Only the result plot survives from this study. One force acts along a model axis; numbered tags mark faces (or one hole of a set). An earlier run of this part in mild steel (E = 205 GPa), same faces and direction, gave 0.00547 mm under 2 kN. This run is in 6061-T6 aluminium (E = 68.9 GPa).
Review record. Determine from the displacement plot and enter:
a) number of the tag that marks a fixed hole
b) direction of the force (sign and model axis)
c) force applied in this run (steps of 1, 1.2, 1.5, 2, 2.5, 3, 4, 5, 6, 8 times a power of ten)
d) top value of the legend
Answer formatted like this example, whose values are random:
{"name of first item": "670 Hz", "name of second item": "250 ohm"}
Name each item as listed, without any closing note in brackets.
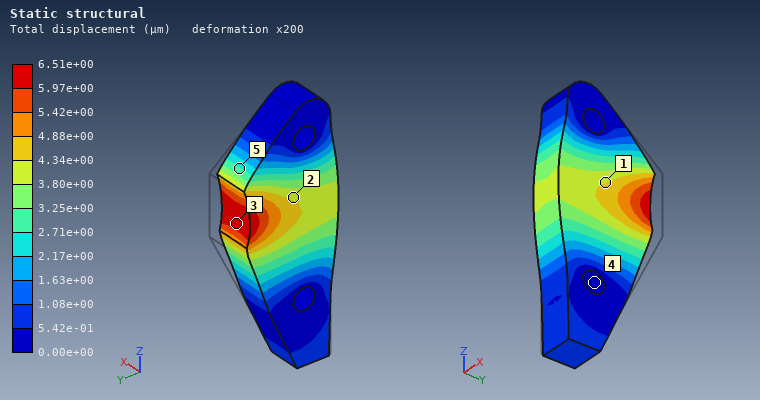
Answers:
{"number of the tag that marks a fixed hole": "4", "direction of the force": "-Y", "force applied in this run": "800 N", "top value of the legend": "6.51e+00 µm"}
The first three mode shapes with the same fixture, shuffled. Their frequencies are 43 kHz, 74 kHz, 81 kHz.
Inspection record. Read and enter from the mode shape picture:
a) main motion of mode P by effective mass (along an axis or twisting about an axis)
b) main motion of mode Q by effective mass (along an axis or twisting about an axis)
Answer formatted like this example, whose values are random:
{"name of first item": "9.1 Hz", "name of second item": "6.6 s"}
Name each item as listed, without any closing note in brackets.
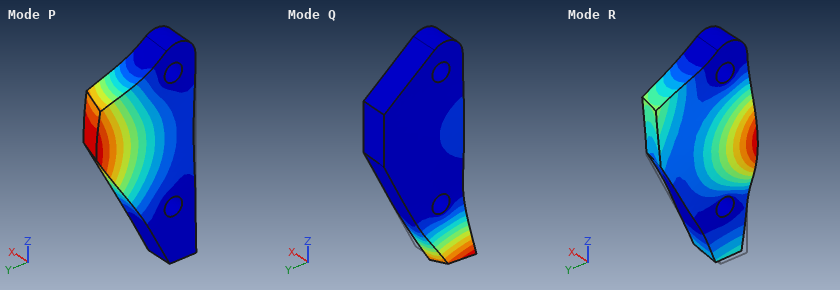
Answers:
{"main motion of mode P by effective mass": "along X", "main motion of mode Q by effective mass": "along X"}
